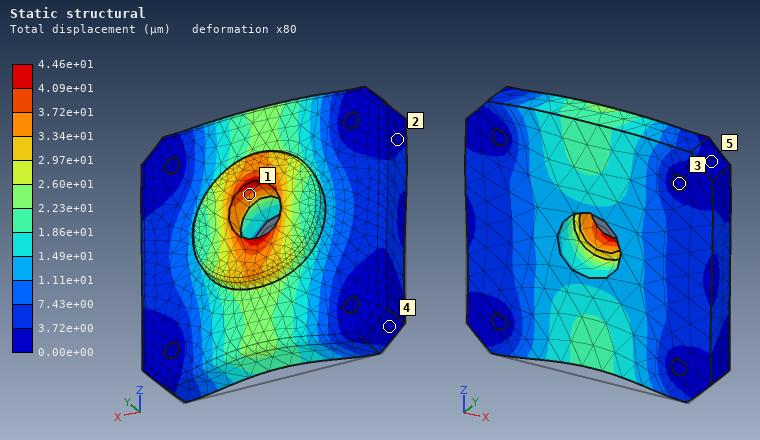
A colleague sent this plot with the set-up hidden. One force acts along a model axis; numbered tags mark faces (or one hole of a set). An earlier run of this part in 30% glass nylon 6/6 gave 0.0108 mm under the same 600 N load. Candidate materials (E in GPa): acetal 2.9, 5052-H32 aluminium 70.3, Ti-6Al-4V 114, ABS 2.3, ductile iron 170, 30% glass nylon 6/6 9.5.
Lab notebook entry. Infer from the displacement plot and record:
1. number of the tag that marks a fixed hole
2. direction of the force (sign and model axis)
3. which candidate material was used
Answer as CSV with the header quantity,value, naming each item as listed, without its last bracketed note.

quantity,value
number of the tag that marks a fixed hole,3
direction of the force,+Z
which candidate material was used,ABS
